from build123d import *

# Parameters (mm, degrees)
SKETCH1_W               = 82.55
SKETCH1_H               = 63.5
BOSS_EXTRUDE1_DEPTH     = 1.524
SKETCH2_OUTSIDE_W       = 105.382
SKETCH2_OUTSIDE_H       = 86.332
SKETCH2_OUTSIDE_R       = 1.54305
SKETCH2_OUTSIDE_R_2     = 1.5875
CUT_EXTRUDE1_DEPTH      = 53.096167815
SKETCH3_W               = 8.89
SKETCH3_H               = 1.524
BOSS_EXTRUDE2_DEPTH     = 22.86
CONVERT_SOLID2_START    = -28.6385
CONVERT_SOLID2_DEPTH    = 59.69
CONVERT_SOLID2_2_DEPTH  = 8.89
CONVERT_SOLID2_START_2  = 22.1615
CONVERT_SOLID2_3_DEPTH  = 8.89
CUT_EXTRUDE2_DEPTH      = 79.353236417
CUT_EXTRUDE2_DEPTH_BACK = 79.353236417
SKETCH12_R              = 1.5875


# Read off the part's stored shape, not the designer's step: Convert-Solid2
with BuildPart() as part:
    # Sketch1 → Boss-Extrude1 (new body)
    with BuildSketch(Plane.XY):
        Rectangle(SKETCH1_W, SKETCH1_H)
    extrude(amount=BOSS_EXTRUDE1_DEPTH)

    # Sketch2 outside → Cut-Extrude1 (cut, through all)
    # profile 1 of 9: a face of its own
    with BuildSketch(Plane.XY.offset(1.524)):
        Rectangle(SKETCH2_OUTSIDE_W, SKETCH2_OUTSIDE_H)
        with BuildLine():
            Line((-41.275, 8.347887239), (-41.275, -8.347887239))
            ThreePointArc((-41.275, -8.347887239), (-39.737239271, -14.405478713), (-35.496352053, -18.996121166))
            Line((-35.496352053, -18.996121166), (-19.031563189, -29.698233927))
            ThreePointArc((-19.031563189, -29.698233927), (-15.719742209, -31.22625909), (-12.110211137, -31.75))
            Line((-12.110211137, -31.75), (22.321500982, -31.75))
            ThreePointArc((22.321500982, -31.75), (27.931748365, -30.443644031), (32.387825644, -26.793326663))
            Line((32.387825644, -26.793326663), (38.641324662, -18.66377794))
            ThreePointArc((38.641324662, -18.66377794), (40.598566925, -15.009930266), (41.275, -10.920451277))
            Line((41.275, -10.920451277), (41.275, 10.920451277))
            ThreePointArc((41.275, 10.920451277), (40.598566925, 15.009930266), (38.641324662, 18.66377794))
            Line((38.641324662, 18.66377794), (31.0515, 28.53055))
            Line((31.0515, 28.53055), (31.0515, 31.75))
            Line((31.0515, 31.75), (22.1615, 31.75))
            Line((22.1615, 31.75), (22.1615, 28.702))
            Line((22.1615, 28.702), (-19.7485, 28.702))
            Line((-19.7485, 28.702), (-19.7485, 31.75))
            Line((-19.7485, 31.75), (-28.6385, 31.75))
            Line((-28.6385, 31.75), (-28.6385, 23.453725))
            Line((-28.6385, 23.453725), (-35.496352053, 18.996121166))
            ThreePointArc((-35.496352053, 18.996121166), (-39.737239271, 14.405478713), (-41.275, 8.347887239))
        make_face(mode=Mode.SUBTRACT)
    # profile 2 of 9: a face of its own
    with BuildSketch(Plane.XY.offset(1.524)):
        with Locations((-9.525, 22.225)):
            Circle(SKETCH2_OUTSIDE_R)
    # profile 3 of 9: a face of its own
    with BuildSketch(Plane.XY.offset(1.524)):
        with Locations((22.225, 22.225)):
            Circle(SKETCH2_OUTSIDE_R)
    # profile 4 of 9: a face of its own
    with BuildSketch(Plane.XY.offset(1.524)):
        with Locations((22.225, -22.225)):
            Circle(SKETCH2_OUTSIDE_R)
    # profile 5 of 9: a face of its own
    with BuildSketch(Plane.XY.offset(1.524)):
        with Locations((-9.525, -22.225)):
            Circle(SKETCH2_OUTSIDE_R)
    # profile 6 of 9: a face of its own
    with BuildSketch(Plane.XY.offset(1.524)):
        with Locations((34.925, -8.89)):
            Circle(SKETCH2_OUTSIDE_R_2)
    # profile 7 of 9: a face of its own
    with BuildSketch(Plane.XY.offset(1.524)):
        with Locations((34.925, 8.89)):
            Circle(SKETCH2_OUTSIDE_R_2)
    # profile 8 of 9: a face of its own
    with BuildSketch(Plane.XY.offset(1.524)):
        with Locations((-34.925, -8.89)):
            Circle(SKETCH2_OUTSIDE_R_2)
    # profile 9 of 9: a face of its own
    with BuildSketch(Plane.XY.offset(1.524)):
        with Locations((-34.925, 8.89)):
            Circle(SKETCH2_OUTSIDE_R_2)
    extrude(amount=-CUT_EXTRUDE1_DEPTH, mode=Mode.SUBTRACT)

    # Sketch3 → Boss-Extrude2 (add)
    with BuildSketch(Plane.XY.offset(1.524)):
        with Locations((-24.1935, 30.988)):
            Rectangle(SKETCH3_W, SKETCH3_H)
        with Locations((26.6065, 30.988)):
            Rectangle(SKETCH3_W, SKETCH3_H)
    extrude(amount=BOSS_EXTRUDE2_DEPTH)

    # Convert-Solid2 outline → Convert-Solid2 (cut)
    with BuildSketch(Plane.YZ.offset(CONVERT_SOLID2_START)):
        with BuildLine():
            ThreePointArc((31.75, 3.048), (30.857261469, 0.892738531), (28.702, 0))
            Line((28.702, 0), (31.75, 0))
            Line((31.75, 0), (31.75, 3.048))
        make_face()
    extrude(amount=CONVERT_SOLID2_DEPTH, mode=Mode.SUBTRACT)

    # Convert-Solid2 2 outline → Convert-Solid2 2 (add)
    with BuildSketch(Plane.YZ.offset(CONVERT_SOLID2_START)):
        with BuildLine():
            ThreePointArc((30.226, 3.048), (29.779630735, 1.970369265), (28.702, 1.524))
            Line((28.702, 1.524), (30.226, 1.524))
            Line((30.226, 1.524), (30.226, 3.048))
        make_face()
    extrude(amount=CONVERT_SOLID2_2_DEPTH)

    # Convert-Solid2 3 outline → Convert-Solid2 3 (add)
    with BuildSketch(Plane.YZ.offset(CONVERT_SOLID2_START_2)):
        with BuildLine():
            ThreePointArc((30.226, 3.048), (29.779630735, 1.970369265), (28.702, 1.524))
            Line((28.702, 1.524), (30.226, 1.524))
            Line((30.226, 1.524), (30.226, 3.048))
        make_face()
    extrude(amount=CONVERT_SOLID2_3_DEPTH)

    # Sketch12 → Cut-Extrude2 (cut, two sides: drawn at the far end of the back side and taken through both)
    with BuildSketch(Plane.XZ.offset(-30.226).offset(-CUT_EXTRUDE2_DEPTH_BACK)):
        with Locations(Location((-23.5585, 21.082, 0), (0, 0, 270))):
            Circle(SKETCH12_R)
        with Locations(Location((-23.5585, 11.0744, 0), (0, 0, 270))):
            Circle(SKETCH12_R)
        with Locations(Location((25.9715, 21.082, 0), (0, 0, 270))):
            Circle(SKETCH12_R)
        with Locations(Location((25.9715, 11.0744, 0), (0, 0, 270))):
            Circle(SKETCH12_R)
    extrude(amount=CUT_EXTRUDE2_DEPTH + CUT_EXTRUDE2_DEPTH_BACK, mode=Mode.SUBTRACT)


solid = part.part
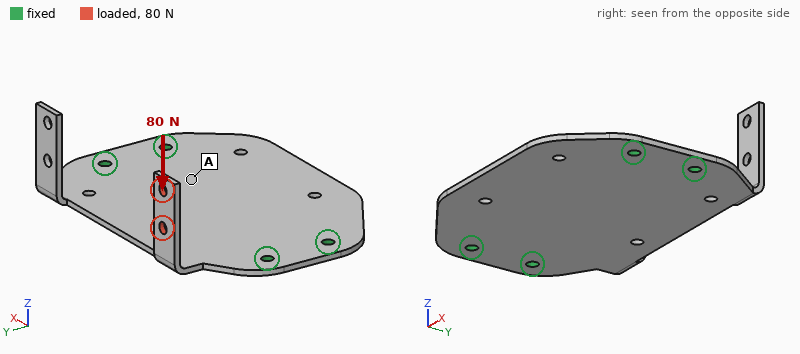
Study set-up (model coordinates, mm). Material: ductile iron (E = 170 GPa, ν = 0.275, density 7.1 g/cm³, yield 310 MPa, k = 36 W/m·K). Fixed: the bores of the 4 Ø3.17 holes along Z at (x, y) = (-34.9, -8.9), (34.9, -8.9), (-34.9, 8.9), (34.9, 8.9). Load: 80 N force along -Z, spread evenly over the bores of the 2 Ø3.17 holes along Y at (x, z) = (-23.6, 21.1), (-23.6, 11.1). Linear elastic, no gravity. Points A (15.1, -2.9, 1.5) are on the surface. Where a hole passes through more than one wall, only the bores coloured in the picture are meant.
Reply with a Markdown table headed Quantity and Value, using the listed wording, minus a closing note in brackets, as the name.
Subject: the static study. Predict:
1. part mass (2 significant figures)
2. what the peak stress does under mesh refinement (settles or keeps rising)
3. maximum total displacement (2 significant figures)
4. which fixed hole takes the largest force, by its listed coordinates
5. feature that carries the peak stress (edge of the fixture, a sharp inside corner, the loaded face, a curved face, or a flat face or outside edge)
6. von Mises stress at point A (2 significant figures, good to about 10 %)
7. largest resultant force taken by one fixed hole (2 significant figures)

| Quantity | Value |
|---|---|
| part mass | 52 g |
| what the peak stress does under mesh refinement | keeps rising |
| maximum total displacement | 0.50 mm |
| which fixed hole takes the largest force, by its listed coordinates | (-34.9, 8.9) |
| feature that carries the peak stress | edge of the fixture |
| von Mises stress at point A | 16 MPa |
| largest resultant force taken by one fixed hole | 100 N |
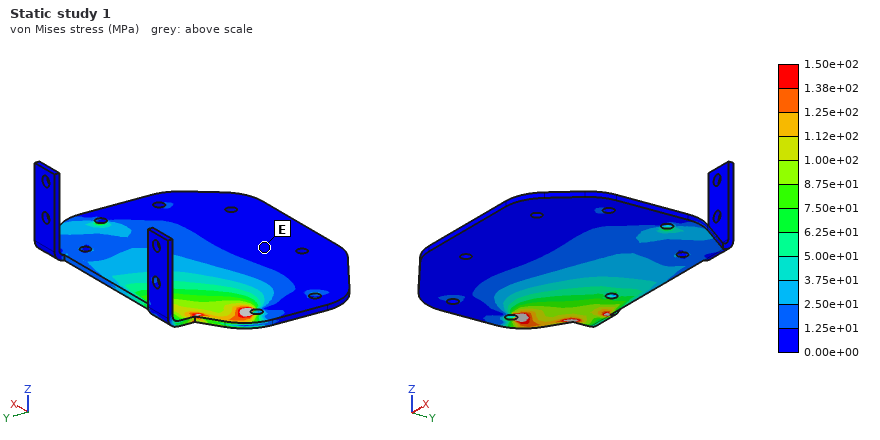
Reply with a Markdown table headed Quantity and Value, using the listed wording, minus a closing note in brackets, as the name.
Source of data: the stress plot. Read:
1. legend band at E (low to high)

| Quantity | Value |
|---|---|
| legend band at E | 0.00e+00 to 1.25e+01 MPa |
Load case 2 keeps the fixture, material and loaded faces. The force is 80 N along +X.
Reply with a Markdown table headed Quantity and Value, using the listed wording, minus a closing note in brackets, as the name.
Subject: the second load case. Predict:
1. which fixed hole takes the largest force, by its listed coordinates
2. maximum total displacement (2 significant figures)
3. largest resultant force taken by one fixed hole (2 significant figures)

| Quantity | Value |
|---|---|
| which fixed hole takes the largest force, by its listed coordinates | (-34.9, 8.9) |
| maximum total displacement | 0.46 mm |
| largest resultant force taken by one fixed hole | 56 N |
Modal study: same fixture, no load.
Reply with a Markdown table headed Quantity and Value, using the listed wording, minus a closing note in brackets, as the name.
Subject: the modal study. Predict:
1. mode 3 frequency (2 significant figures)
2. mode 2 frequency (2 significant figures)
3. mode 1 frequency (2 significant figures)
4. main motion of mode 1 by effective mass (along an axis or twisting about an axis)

| Quantity | Value |
|---|---|
| mode 3 frequency | 1300 Hz |
| mode 2 frequency | 1200 Hz |
| mode 1 frequency | 1000 Hz |
| main motion of mode 1 by effective mass | along Z |
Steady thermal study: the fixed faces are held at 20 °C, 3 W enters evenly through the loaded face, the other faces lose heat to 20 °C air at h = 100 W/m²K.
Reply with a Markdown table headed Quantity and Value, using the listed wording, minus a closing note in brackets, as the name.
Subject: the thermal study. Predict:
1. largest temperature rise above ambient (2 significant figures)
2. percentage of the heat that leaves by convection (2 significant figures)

| Quantity | Value |
|---|---|
| largest temperature rise above ambient | 62 K |
| percentage of the heat that leaves by convection | 92 % |
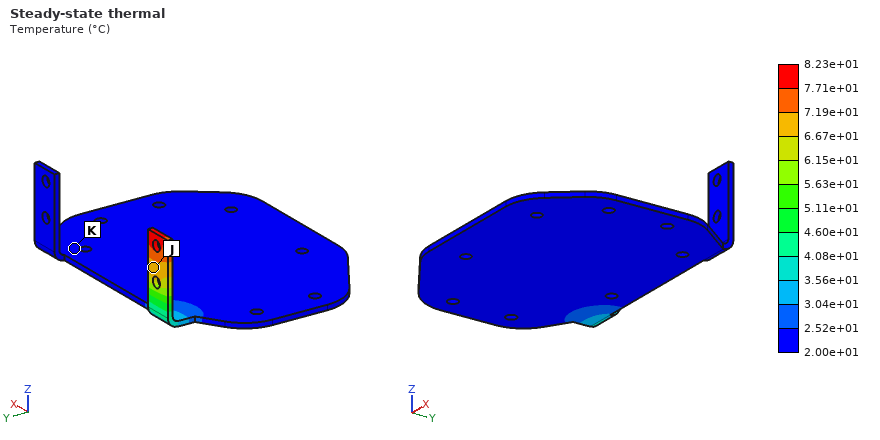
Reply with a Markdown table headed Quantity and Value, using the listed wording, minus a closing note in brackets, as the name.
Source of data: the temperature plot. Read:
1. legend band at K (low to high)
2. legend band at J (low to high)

| Quantity | Value |
|---|---|
| legend band at K | 2.00e+01 to 2.52e+01 °C |
| legend band at J | 6.67e+01 to 7.19e+01 °C |
